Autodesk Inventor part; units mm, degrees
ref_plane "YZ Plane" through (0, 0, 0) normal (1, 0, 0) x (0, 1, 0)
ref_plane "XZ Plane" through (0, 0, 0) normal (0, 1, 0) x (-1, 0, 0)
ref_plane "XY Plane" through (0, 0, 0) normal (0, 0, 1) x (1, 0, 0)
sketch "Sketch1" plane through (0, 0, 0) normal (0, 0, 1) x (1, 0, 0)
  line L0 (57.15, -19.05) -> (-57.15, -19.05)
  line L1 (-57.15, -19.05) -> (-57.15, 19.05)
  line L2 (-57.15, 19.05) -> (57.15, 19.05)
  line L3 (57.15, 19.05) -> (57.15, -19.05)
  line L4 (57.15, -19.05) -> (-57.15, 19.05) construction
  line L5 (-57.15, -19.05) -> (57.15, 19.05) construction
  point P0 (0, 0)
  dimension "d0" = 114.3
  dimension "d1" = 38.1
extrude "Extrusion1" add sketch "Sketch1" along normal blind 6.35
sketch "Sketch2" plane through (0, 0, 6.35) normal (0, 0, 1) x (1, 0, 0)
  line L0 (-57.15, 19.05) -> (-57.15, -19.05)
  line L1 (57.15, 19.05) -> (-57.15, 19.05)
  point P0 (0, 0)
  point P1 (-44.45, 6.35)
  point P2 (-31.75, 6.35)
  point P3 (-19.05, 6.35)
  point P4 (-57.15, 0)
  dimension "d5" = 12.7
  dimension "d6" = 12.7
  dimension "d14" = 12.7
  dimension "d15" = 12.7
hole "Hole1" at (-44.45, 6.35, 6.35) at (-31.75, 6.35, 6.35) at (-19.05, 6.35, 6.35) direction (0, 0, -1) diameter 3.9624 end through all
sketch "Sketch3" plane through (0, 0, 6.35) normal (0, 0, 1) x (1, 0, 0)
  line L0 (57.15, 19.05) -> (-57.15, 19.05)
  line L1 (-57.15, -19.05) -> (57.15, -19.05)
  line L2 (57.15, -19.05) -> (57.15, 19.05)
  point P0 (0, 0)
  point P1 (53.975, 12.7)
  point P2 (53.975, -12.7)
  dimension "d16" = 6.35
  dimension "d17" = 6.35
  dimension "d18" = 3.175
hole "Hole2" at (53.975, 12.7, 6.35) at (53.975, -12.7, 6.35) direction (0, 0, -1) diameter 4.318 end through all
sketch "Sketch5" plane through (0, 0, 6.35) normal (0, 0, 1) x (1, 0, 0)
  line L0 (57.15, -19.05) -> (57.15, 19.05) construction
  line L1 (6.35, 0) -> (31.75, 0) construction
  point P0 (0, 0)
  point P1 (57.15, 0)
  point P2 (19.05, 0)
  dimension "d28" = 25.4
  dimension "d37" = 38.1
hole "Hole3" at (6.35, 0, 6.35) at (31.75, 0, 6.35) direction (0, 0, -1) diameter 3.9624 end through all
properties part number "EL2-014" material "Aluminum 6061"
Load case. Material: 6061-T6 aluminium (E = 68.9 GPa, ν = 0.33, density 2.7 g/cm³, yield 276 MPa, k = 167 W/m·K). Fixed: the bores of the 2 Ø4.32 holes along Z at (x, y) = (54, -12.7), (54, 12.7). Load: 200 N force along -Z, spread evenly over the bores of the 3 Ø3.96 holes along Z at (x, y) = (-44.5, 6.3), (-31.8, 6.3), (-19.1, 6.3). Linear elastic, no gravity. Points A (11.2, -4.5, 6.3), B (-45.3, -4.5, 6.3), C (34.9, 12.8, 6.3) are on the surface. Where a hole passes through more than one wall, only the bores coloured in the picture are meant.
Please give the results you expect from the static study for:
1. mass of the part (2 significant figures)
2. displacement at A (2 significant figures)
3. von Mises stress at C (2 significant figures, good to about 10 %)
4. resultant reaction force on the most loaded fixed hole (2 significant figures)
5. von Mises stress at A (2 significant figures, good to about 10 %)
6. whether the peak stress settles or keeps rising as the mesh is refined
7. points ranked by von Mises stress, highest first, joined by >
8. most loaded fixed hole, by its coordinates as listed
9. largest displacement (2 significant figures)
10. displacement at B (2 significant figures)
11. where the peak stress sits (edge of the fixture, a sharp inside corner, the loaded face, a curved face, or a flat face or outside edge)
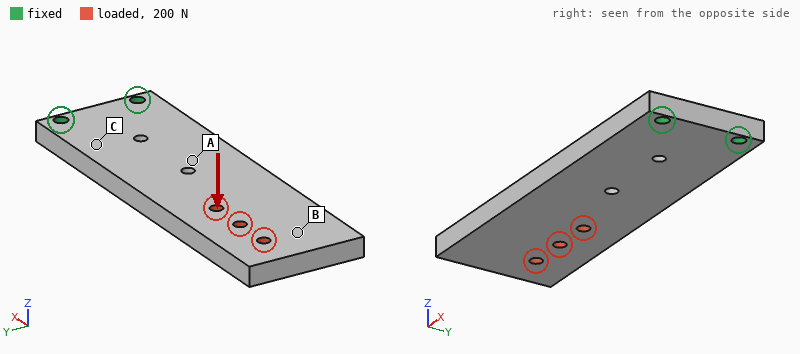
73 g
0.26 mm
55 MPa
140 N
34 MPa
keeps rising
C > A > B
(54, 12.7)
1.2 mm
0.98 mm
edge of the fixture
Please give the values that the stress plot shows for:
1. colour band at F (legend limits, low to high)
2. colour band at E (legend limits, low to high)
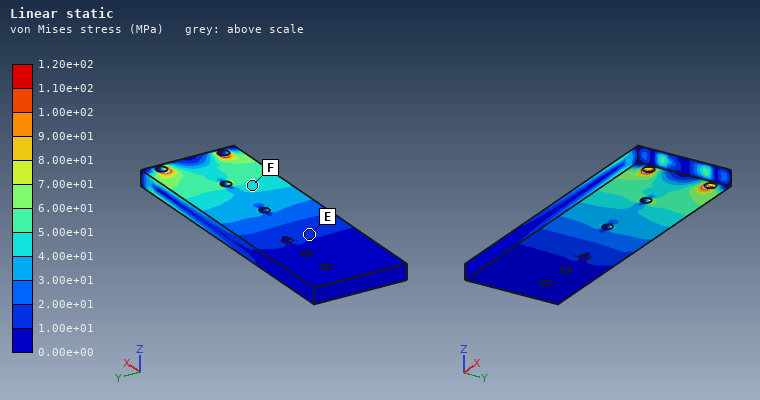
4.00e+01 to 5.00e+01 MPa
1.00e+01 to 2.00e+01 MPa
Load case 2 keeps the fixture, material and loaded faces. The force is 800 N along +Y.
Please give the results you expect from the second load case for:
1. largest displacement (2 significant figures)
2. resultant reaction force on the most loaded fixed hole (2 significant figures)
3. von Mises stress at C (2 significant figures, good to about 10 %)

0.14 mm
2.5 kN
24 MPa
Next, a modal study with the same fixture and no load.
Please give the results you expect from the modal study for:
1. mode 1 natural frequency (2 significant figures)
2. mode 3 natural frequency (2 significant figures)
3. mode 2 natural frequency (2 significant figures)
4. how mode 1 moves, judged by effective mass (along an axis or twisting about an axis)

410 Hz
2300 Hz
2300 Hz
along Z
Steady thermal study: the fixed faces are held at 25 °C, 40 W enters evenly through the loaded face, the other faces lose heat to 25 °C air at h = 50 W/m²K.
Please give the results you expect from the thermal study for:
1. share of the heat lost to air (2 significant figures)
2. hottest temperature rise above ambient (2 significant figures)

43 %
60 K
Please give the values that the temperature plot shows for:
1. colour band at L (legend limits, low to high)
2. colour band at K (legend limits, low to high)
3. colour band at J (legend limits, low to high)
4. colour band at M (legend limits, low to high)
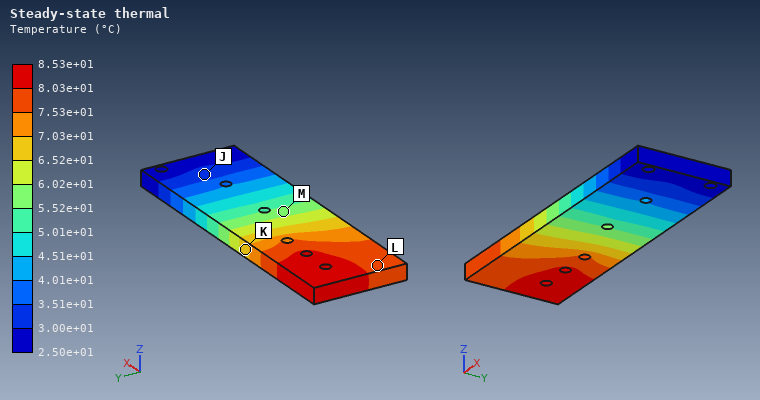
7.53e+01 to 8.03e+01 °C
6.52e+01 to 7.03e+01 °C
3.00e+01 to 3.51e+01 °C
5.52e+01 to 6.02e+01 °C
